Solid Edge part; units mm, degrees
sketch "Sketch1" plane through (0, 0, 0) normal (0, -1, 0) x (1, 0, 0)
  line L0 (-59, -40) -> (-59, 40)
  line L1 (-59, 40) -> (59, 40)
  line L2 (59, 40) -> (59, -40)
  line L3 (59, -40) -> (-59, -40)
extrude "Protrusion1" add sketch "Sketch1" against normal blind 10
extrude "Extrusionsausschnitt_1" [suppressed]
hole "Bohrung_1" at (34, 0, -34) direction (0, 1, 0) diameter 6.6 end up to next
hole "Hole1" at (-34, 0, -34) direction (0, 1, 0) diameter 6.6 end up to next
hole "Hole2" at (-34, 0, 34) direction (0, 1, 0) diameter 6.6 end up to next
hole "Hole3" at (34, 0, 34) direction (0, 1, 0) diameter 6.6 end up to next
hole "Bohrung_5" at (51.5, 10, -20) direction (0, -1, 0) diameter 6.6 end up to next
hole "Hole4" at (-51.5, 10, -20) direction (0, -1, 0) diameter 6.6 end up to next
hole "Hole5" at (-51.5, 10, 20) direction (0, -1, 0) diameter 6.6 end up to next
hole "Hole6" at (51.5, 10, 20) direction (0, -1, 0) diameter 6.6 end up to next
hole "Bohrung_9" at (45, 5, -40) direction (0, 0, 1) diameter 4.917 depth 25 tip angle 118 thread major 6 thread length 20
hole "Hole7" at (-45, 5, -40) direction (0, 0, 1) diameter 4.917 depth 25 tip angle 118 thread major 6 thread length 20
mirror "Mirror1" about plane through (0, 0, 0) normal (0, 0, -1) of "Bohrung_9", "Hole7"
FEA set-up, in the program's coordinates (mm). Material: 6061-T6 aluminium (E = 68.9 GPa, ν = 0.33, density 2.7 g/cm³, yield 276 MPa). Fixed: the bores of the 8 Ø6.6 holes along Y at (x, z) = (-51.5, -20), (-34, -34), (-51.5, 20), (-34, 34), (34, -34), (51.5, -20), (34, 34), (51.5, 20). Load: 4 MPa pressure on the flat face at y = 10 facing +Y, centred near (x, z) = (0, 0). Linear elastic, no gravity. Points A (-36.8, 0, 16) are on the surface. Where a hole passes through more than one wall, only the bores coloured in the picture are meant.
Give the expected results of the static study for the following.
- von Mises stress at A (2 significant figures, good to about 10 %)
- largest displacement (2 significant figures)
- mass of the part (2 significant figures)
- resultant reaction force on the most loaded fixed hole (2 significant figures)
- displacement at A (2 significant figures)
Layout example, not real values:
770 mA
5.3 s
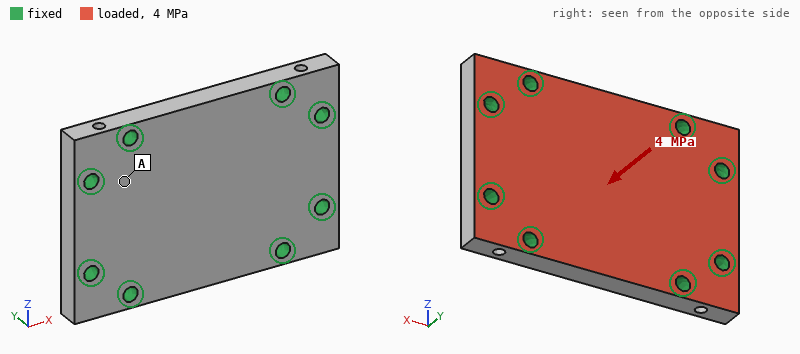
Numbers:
32 MPa
98 µm
240 g
6.1 kN
25 µm
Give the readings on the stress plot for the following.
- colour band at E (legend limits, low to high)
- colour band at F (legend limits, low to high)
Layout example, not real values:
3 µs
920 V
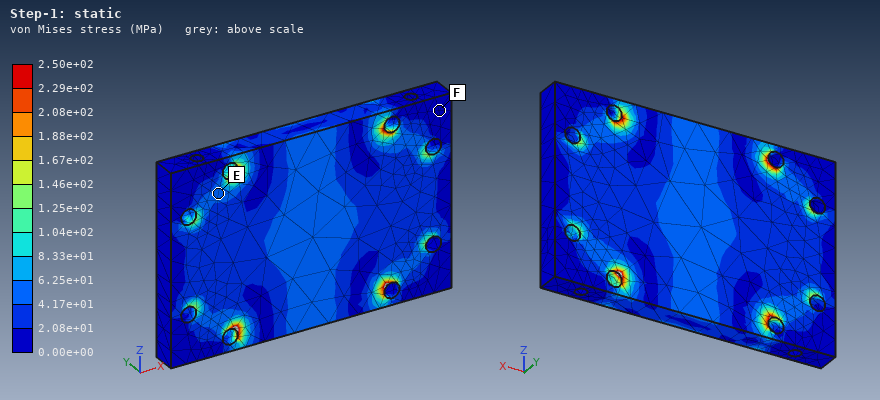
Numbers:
4.17e+01 to 6.25e+01 MPa
0.00e+00 to 2.08e+01 MPa
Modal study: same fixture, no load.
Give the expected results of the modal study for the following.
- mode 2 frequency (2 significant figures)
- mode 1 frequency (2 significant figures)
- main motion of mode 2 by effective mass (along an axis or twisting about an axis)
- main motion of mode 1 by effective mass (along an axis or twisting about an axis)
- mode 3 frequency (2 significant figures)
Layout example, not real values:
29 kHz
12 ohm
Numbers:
11 kHz
7500 Hz
twisting about X
along Y
15 kHz
